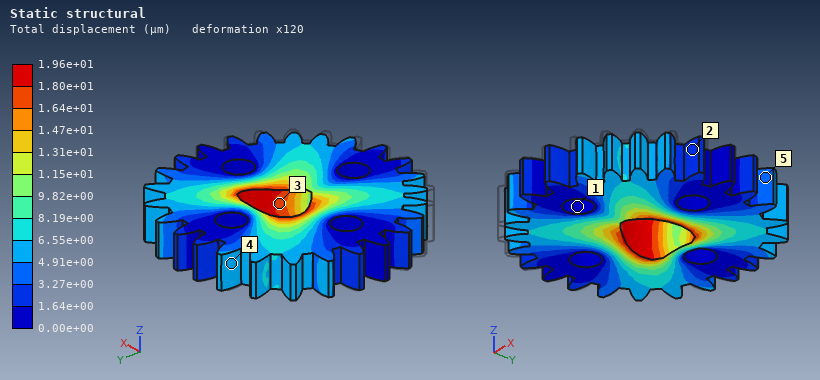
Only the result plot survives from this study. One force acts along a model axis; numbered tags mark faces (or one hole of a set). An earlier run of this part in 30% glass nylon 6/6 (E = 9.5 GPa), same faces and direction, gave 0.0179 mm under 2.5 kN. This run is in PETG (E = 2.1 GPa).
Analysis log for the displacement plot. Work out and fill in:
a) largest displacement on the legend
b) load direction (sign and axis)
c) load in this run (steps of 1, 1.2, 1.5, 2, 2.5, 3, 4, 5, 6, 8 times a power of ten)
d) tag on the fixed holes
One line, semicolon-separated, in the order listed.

1.96e+01 µm; +Y; 600 N; 1
